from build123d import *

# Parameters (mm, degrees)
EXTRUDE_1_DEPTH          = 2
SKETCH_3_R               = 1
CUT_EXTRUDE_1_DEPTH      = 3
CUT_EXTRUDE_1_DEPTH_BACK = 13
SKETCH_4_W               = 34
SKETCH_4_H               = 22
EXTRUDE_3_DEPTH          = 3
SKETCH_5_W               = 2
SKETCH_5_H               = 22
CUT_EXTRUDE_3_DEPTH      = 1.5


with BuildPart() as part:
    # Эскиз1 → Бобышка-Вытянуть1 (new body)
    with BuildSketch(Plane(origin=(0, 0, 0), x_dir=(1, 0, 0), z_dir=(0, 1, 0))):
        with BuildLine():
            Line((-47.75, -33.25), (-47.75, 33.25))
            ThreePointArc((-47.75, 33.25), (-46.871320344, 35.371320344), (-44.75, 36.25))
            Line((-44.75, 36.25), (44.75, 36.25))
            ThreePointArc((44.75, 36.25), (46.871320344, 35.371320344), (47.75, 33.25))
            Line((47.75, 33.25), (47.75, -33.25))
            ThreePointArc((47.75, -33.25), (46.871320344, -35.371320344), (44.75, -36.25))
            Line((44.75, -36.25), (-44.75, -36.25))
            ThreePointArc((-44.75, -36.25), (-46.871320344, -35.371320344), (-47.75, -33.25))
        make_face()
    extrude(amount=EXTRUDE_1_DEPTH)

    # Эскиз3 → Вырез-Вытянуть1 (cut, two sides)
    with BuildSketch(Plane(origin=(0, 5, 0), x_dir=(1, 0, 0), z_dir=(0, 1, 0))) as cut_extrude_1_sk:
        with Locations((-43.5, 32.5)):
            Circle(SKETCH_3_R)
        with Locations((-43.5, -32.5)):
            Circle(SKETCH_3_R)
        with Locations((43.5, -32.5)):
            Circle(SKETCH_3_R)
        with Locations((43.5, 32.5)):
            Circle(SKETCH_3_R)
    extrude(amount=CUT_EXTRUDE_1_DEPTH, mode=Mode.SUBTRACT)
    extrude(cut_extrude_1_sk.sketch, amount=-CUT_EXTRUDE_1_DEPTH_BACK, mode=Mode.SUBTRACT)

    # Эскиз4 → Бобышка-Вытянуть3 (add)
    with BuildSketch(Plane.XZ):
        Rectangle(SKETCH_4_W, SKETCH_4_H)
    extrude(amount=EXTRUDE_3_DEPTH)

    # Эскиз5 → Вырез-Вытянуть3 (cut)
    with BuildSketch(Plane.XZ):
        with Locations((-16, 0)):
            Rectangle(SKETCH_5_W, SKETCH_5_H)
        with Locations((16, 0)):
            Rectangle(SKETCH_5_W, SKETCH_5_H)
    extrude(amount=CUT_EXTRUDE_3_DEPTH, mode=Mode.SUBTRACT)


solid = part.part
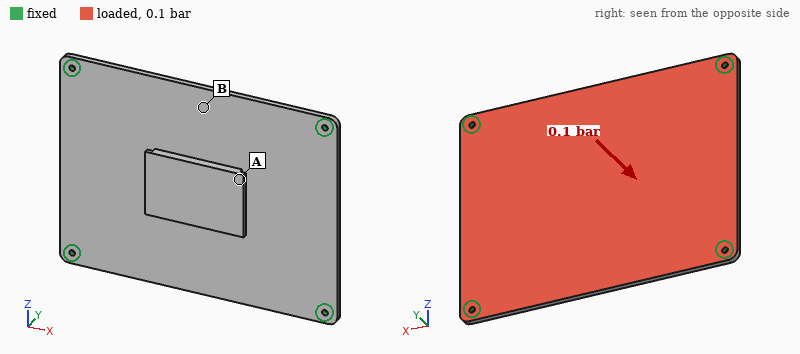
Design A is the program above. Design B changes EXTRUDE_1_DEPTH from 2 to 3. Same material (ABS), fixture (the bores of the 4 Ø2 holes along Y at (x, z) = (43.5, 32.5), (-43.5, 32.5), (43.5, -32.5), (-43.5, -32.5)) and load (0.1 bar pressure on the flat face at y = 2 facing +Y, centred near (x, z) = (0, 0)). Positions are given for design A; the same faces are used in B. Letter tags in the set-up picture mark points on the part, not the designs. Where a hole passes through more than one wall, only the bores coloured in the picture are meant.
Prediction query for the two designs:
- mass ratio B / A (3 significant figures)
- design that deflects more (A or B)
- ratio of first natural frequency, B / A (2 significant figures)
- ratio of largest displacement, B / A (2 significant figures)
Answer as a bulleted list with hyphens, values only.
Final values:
- 1.43
- A
- 1.5
- 0.33
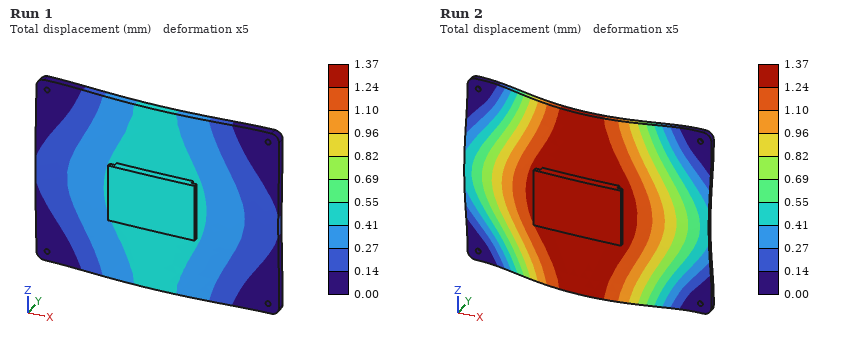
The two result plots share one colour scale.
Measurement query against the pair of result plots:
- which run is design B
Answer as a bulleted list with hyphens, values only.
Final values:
- Run 1
